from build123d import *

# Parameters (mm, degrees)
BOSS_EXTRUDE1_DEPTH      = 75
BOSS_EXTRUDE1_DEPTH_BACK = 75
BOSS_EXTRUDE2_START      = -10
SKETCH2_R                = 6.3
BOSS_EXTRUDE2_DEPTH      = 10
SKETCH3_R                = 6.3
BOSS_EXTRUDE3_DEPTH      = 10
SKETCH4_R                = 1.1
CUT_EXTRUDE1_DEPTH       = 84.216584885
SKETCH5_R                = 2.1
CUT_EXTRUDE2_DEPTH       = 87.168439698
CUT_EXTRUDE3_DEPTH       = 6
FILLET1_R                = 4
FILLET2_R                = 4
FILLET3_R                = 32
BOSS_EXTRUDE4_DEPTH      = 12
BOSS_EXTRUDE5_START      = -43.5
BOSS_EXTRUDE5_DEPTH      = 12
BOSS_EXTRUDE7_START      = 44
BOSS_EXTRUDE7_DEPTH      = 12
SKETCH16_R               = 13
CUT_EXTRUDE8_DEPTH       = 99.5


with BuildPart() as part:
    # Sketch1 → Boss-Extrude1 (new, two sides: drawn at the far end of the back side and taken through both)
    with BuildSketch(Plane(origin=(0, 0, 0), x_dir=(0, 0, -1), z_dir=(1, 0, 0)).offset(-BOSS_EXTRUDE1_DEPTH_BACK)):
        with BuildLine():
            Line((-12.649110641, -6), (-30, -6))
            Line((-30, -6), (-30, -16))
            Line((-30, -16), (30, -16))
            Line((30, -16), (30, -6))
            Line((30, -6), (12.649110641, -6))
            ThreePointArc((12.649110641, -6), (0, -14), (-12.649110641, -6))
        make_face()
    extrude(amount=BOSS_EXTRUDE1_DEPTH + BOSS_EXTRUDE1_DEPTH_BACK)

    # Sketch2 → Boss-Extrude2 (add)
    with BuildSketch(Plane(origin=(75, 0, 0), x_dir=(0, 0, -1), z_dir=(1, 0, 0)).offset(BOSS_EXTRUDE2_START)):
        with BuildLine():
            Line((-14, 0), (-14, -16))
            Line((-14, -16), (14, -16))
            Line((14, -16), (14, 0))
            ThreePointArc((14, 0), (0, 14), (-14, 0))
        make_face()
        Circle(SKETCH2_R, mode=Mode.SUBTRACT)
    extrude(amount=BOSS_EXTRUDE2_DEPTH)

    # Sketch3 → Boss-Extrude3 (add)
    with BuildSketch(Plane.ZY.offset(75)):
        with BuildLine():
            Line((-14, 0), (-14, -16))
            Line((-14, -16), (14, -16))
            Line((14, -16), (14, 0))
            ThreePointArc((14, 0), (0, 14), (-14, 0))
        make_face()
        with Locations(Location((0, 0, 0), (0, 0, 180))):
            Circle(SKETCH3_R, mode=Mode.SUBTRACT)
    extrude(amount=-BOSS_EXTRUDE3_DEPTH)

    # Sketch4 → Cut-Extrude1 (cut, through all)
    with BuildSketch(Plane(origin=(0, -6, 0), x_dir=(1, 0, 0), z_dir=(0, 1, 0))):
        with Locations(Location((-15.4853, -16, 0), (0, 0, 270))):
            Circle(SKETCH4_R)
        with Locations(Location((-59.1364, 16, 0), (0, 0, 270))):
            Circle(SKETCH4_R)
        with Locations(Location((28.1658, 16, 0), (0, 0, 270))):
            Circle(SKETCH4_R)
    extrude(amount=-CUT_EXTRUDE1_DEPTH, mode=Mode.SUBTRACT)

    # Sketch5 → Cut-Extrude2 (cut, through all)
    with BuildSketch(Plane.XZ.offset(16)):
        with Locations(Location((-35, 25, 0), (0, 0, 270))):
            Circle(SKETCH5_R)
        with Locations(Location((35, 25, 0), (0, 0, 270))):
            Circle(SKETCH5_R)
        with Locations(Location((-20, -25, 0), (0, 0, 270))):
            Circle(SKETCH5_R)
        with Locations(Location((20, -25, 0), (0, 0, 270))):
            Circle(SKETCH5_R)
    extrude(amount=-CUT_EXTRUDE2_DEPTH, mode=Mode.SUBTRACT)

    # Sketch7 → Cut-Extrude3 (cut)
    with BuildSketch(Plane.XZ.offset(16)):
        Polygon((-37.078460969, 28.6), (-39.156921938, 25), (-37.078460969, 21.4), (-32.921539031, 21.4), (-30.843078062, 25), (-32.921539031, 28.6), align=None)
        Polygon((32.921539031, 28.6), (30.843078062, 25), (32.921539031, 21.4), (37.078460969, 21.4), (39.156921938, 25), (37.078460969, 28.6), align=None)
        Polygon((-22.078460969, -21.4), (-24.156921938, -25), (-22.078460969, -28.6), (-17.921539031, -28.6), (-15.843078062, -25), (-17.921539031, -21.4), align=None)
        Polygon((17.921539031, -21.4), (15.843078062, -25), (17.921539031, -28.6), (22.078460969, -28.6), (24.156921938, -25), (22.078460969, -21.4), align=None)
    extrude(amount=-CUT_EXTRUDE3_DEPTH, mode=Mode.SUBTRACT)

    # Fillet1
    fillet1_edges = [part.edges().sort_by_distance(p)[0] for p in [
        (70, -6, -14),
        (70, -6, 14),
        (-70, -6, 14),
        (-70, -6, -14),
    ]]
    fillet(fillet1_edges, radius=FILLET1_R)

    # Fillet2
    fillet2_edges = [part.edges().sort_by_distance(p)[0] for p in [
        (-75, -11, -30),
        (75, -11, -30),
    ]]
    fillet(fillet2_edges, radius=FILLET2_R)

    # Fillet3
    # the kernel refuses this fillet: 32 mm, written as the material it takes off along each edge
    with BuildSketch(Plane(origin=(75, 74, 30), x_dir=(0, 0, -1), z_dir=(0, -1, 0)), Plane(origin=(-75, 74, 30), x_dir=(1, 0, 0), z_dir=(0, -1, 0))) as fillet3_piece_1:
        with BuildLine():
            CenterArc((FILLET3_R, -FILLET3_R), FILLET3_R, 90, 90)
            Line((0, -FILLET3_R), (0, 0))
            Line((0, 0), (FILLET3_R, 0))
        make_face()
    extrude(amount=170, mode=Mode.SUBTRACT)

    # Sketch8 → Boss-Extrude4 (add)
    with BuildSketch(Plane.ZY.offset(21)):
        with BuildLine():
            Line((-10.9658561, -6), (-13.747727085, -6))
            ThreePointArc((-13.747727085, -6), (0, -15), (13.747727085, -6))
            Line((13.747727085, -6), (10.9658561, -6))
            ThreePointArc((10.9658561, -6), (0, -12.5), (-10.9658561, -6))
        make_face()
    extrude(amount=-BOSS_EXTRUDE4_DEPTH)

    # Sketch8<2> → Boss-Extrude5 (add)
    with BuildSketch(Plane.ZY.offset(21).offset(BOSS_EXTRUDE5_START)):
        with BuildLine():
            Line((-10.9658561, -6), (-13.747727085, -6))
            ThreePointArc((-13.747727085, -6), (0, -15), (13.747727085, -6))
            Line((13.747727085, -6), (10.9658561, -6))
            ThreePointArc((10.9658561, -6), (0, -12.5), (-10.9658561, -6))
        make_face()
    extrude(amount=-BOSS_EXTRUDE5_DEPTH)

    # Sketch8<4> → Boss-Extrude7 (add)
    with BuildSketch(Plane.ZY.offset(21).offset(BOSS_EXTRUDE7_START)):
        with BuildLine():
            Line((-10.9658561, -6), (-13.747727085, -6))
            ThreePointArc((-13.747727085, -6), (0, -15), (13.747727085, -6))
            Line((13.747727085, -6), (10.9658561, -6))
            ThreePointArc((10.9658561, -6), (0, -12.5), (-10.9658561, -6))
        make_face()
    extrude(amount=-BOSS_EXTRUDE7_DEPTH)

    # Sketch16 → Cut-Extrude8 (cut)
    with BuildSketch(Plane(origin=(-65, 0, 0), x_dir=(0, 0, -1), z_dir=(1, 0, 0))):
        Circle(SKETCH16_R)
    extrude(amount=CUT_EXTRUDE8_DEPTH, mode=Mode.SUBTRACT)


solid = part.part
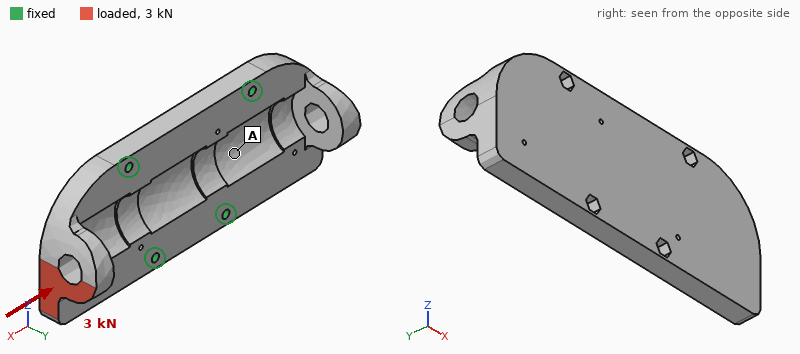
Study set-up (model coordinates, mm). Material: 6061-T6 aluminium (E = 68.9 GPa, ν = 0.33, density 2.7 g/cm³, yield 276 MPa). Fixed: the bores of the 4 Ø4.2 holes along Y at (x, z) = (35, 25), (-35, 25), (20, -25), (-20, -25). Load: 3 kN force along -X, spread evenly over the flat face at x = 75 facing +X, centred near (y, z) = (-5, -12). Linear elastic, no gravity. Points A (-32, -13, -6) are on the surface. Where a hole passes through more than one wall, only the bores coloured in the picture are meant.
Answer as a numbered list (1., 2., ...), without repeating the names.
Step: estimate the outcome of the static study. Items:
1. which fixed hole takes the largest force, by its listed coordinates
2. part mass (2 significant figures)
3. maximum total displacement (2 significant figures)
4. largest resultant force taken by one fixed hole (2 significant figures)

1. (20, -25)
2. 200 g
3. 0.19 mm
4. 2.1 kN
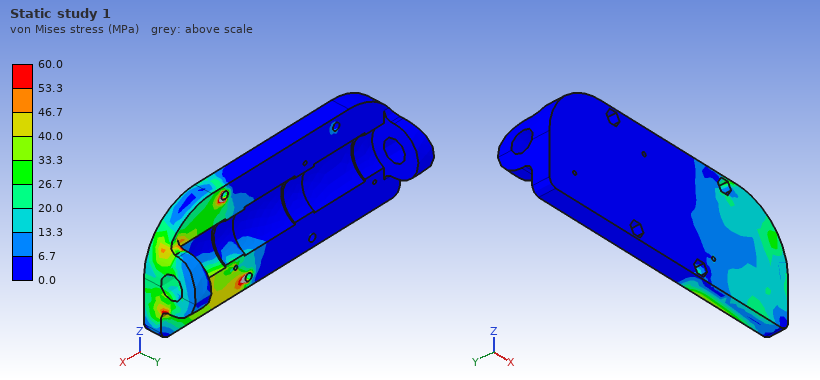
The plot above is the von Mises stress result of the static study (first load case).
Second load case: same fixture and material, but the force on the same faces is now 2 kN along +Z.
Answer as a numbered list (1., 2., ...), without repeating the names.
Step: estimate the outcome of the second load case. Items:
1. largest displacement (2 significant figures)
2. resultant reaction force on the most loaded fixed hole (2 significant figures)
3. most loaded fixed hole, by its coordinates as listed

1. 85 µm
2. 2.0 kN
3. (35, 25)
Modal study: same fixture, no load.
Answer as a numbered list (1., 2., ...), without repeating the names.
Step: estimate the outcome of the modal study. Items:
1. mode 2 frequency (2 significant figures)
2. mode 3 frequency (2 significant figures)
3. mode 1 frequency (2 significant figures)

1. 2100 Hz
2. 4700 Hz
3. 2100 Hz
